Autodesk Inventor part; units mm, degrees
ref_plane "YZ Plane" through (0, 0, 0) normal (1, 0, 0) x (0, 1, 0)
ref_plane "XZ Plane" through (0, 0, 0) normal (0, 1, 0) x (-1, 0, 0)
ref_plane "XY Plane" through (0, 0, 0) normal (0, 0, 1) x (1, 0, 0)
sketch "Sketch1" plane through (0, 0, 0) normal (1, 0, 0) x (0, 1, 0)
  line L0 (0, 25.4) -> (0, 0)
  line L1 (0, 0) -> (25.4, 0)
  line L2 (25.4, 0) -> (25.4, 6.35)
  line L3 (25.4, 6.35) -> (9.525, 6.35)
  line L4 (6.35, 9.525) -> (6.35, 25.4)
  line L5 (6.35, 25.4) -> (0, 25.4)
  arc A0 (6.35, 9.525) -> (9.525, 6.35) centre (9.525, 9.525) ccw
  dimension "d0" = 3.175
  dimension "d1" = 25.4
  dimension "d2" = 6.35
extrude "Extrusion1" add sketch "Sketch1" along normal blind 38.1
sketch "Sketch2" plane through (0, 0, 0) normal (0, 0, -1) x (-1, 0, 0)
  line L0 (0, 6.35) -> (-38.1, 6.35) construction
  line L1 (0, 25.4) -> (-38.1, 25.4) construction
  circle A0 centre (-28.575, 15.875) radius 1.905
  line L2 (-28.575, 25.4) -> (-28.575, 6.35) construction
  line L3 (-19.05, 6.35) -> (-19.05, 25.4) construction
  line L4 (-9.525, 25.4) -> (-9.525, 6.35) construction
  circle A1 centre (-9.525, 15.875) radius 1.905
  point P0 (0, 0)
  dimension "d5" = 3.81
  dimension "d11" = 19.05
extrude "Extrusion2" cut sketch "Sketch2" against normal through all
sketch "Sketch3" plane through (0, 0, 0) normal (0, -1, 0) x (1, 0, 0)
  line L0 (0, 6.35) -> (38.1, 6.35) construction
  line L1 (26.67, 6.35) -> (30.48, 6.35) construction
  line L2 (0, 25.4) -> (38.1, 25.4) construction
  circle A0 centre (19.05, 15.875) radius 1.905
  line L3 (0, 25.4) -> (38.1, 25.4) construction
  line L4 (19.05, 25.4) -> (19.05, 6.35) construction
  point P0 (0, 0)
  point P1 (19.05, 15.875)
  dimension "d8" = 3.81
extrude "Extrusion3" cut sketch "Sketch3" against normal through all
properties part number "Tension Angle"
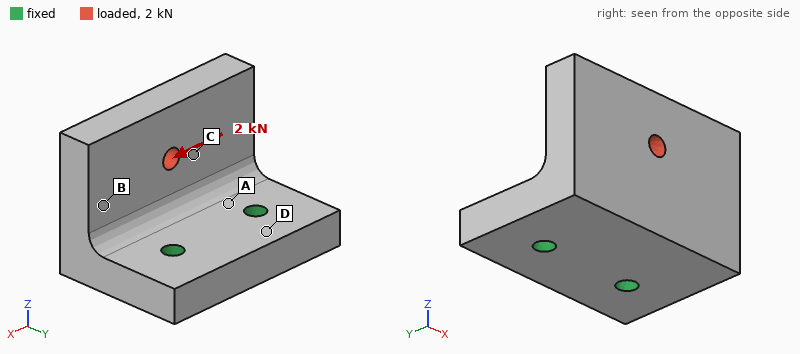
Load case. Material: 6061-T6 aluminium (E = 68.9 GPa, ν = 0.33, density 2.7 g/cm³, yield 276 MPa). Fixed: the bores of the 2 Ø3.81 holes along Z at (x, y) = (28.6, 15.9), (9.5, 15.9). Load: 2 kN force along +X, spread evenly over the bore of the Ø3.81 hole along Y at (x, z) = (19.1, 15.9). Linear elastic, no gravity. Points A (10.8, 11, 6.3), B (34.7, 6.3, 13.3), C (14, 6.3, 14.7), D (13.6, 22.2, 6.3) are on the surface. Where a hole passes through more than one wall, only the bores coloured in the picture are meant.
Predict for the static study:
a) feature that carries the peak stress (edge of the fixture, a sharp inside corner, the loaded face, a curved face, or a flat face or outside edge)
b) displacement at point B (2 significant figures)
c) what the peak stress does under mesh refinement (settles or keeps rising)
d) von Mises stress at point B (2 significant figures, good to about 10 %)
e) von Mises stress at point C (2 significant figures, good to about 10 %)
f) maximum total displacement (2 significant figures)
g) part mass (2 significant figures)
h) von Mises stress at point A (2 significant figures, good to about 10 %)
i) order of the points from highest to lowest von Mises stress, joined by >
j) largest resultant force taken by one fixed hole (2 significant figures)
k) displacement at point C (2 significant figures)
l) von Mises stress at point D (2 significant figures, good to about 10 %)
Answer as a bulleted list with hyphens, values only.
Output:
- edge of the fixture
- 29 µm
- keeps rising
- 20 MPa
- 32 MPa
- 48 µm
- 29 g
- 50 MPa
- A > C > B > D
- 1.8 kN
- 25 µm
- 8.9 MPa
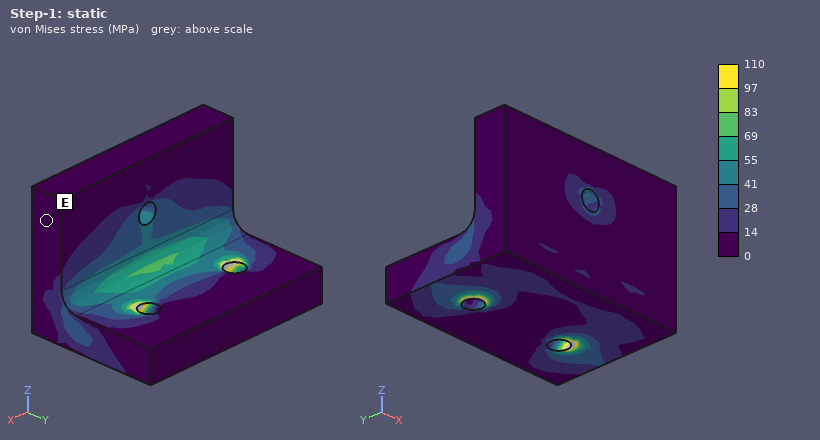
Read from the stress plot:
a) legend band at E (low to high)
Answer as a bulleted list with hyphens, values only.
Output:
- 0 to 14 MPa
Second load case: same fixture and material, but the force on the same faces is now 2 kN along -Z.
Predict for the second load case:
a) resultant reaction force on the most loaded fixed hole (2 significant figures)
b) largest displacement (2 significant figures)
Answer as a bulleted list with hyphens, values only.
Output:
- 1.0 kN
- 85 µm
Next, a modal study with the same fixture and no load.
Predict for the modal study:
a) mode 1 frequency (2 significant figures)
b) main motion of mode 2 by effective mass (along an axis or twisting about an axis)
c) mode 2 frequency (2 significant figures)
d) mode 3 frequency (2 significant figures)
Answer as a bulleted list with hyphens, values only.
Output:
- 5600 Hz
- along X
- 9300 Hz
- 15 kHz
